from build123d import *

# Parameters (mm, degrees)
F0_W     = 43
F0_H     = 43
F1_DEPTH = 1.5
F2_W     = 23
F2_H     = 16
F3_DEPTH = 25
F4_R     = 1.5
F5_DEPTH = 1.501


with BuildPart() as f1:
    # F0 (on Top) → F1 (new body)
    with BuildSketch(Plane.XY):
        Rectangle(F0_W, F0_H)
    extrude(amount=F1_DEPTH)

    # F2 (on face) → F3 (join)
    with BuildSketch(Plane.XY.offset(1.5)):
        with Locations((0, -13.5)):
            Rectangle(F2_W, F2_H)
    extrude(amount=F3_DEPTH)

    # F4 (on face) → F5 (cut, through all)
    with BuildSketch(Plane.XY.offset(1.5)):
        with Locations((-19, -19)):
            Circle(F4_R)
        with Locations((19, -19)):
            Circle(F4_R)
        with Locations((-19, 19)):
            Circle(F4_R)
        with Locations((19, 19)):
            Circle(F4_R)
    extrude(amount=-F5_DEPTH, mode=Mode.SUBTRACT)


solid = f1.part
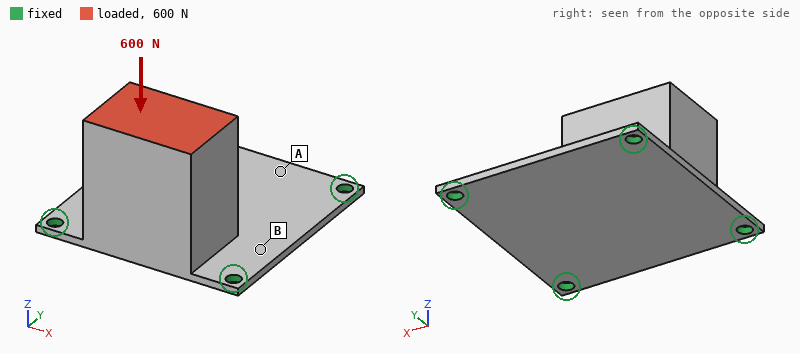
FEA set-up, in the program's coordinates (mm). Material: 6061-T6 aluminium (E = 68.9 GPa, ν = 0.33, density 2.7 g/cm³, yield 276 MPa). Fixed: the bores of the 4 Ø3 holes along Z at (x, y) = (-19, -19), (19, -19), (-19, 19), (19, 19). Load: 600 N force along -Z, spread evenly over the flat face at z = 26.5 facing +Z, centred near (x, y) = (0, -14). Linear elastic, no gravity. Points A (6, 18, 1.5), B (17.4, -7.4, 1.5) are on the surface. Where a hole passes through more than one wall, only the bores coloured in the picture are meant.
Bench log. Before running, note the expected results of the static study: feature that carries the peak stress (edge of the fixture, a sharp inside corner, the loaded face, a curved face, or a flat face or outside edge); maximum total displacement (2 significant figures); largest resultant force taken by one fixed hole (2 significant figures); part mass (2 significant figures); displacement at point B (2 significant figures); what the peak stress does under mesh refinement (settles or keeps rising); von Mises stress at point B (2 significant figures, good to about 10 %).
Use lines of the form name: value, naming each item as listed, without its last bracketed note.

feature that carries the peak stress: edge of the fixture
maximum total displacement: 0.15 mm
largest resultant force taken by one fixed hole: 290 N
part mass: 32 g
displacement at point B: 0.071 mm
what the peak stress does under mesh refinement: keeps rising
von Mises stress at point B: 44 MPa
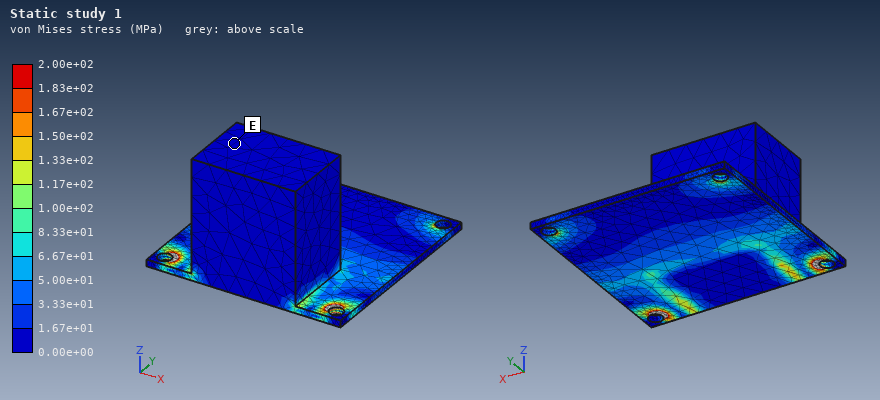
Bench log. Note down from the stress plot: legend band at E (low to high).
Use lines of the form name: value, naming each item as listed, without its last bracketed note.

legend band at E: 0.00e+00 to 1.67e+01 MPa
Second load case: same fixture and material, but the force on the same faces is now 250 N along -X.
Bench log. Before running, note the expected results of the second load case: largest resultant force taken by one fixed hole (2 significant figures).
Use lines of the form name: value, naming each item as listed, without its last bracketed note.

largest resultant force taken by one fixed hole: 230 N
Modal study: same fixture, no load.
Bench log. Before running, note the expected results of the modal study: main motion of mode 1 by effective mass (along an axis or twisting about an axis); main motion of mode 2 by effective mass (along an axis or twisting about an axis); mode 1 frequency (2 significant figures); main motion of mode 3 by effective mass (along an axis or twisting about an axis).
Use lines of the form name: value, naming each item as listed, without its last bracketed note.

main motion of mode 1 by effective mass: along Y
main motion of mode 2 by effective mass: along X
mode 1 frequency: 1200 Hz
main motion of mode 3 by effective mass: along Z
